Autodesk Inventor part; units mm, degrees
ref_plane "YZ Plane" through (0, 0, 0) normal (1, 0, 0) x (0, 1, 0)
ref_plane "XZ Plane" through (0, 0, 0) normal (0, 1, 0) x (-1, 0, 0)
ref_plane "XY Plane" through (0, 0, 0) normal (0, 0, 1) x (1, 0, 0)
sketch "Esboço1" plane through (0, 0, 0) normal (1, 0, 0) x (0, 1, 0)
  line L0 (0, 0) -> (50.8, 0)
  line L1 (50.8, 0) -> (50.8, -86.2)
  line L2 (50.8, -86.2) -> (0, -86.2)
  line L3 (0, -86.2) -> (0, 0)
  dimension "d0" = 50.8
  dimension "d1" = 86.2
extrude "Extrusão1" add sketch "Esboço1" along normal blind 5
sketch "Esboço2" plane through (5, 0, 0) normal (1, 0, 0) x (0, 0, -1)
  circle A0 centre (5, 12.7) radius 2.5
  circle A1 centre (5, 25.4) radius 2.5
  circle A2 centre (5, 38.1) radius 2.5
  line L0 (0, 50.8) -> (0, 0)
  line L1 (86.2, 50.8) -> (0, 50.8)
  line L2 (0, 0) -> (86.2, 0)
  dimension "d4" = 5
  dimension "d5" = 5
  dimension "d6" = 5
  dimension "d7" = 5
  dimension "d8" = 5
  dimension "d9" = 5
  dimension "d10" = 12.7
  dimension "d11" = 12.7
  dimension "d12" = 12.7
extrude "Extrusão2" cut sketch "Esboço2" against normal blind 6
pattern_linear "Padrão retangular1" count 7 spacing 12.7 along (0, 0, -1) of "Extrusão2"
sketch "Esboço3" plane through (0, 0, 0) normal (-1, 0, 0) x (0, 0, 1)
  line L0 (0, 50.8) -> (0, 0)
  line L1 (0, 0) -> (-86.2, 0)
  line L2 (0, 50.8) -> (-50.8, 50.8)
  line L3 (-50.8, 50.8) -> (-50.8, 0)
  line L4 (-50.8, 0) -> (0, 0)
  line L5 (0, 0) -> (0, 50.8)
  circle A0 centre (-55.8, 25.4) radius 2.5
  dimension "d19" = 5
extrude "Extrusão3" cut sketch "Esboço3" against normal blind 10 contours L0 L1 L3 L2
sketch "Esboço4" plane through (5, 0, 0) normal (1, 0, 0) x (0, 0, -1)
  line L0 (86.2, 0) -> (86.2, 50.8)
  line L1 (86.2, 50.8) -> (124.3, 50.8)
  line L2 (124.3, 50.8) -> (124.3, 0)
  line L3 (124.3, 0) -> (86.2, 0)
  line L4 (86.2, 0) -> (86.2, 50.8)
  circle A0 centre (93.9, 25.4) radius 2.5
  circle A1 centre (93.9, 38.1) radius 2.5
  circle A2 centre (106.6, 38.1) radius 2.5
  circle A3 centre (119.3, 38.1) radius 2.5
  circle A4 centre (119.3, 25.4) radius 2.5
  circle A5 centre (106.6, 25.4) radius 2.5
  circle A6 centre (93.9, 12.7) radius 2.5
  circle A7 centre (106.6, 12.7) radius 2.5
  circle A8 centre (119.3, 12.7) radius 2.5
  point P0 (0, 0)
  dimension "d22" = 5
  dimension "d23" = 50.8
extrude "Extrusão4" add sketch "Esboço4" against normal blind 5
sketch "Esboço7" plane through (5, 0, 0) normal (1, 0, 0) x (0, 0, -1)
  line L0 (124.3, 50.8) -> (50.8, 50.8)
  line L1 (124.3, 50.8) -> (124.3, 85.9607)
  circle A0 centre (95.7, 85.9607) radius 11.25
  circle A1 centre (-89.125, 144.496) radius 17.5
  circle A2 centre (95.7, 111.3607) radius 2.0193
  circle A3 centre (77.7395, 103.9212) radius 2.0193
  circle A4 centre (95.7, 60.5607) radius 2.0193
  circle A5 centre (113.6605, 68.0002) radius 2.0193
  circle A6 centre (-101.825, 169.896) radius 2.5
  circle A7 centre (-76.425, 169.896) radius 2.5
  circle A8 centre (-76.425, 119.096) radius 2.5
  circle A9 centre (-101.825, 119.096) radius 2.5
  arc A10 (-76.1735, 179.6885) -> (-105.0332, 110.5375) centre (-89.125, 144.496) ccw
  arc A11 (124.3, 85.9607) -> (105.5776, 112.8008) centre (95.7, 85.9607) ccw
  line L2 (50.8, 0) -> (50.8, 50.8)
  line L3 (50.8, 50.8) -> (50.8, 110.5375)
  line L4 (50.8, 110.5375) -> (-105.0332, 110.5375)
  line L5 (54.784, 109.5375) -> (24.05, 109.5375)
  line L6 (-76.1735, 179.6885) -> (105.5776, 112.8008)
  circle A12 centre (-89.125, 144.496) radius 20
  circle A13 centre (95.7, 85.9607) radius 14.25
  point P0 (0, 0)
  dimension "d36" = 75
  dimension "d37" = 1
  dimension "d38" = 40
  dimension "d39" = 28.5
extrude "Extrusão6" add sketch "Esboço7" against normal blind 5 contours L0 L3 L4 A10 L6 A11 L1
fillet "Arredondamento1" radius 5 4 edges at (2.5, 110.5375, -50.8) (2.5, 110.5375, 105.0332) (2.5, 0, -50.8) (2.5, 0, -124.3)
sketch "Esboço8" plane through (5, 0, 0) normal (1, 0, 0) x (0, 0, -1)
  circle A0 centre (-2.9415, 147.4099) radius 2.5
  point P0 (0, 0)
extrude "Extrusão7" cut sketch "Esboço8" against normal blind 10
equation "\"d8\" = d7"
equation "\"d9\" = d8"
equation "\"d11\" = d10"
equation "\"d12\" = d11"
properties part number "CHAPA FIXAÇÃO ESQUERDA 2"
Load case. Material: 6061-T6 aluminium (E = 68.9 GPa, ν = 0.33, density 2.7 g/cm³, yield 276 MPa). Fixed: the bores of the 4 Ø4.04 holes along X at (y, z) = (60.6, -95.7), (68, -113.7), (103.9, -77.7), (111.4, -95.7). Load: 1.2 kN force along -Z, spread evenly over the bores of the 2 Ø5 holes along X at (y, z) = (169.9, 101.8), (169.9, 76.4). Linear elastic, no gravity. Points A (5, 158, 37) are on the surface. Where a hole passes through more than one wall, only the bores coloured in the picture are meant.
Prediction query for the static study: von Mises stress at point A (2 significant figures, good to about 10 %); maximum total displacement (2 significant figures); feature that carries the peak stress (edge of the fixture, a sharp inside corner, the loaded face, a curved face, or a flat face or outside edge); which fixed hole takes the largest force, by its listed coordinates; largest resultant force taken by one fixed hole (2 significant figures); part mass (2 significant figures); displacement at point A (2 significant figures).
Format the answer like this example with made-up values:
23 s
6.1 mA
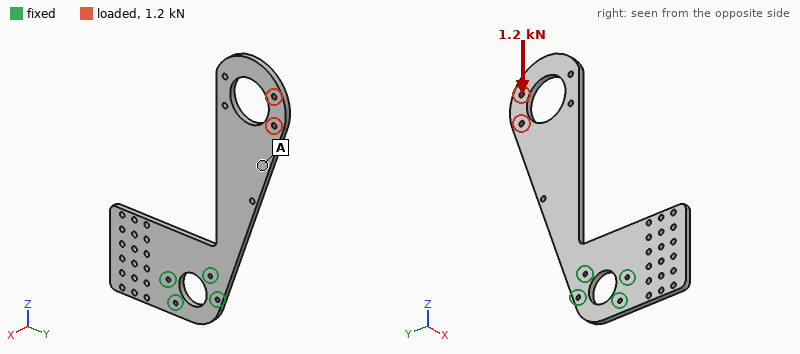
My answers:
17 MPa
1.4 mm
a curved face
(111.4, -95.7)
2.0 kN
210 g
0.73 mm
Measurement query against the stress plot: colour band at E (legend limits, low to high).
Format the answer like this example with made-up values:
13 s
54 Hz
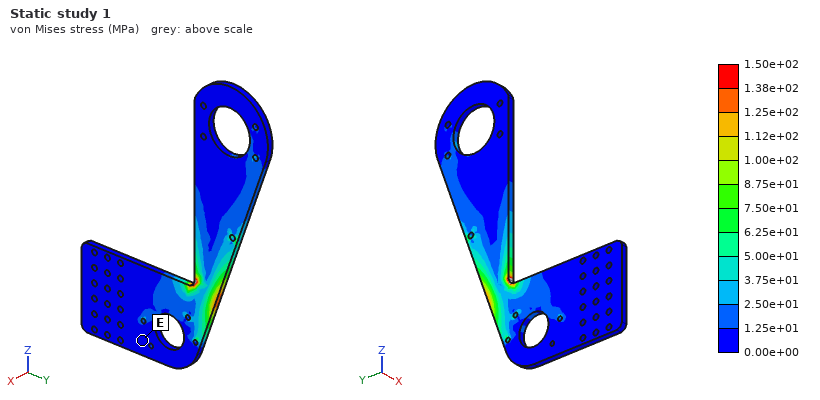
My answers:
0.00e+00 to 1.25e+01 MPa
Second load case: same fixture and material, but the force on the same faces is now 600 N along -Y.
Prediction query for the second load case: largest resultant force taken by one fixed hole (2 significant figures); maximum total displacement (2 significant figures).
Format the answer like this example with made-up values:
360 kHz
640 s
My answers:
2.2 kN
1.9 mm
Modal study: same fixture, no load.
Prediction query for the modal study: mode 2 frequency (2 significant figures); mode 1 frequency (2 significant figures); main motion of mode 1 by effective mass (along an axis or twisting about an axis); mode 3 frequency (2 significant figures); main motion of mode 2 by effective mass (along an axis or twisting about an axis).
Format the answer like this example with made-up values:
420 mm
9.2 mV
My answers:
420 Hz
79 Hz
along X
460 Hz
along Y
